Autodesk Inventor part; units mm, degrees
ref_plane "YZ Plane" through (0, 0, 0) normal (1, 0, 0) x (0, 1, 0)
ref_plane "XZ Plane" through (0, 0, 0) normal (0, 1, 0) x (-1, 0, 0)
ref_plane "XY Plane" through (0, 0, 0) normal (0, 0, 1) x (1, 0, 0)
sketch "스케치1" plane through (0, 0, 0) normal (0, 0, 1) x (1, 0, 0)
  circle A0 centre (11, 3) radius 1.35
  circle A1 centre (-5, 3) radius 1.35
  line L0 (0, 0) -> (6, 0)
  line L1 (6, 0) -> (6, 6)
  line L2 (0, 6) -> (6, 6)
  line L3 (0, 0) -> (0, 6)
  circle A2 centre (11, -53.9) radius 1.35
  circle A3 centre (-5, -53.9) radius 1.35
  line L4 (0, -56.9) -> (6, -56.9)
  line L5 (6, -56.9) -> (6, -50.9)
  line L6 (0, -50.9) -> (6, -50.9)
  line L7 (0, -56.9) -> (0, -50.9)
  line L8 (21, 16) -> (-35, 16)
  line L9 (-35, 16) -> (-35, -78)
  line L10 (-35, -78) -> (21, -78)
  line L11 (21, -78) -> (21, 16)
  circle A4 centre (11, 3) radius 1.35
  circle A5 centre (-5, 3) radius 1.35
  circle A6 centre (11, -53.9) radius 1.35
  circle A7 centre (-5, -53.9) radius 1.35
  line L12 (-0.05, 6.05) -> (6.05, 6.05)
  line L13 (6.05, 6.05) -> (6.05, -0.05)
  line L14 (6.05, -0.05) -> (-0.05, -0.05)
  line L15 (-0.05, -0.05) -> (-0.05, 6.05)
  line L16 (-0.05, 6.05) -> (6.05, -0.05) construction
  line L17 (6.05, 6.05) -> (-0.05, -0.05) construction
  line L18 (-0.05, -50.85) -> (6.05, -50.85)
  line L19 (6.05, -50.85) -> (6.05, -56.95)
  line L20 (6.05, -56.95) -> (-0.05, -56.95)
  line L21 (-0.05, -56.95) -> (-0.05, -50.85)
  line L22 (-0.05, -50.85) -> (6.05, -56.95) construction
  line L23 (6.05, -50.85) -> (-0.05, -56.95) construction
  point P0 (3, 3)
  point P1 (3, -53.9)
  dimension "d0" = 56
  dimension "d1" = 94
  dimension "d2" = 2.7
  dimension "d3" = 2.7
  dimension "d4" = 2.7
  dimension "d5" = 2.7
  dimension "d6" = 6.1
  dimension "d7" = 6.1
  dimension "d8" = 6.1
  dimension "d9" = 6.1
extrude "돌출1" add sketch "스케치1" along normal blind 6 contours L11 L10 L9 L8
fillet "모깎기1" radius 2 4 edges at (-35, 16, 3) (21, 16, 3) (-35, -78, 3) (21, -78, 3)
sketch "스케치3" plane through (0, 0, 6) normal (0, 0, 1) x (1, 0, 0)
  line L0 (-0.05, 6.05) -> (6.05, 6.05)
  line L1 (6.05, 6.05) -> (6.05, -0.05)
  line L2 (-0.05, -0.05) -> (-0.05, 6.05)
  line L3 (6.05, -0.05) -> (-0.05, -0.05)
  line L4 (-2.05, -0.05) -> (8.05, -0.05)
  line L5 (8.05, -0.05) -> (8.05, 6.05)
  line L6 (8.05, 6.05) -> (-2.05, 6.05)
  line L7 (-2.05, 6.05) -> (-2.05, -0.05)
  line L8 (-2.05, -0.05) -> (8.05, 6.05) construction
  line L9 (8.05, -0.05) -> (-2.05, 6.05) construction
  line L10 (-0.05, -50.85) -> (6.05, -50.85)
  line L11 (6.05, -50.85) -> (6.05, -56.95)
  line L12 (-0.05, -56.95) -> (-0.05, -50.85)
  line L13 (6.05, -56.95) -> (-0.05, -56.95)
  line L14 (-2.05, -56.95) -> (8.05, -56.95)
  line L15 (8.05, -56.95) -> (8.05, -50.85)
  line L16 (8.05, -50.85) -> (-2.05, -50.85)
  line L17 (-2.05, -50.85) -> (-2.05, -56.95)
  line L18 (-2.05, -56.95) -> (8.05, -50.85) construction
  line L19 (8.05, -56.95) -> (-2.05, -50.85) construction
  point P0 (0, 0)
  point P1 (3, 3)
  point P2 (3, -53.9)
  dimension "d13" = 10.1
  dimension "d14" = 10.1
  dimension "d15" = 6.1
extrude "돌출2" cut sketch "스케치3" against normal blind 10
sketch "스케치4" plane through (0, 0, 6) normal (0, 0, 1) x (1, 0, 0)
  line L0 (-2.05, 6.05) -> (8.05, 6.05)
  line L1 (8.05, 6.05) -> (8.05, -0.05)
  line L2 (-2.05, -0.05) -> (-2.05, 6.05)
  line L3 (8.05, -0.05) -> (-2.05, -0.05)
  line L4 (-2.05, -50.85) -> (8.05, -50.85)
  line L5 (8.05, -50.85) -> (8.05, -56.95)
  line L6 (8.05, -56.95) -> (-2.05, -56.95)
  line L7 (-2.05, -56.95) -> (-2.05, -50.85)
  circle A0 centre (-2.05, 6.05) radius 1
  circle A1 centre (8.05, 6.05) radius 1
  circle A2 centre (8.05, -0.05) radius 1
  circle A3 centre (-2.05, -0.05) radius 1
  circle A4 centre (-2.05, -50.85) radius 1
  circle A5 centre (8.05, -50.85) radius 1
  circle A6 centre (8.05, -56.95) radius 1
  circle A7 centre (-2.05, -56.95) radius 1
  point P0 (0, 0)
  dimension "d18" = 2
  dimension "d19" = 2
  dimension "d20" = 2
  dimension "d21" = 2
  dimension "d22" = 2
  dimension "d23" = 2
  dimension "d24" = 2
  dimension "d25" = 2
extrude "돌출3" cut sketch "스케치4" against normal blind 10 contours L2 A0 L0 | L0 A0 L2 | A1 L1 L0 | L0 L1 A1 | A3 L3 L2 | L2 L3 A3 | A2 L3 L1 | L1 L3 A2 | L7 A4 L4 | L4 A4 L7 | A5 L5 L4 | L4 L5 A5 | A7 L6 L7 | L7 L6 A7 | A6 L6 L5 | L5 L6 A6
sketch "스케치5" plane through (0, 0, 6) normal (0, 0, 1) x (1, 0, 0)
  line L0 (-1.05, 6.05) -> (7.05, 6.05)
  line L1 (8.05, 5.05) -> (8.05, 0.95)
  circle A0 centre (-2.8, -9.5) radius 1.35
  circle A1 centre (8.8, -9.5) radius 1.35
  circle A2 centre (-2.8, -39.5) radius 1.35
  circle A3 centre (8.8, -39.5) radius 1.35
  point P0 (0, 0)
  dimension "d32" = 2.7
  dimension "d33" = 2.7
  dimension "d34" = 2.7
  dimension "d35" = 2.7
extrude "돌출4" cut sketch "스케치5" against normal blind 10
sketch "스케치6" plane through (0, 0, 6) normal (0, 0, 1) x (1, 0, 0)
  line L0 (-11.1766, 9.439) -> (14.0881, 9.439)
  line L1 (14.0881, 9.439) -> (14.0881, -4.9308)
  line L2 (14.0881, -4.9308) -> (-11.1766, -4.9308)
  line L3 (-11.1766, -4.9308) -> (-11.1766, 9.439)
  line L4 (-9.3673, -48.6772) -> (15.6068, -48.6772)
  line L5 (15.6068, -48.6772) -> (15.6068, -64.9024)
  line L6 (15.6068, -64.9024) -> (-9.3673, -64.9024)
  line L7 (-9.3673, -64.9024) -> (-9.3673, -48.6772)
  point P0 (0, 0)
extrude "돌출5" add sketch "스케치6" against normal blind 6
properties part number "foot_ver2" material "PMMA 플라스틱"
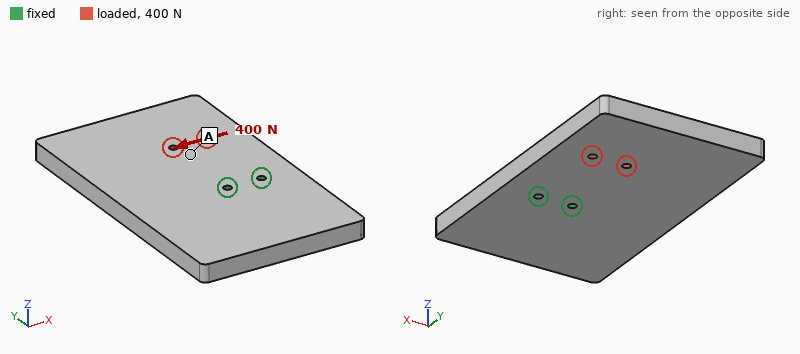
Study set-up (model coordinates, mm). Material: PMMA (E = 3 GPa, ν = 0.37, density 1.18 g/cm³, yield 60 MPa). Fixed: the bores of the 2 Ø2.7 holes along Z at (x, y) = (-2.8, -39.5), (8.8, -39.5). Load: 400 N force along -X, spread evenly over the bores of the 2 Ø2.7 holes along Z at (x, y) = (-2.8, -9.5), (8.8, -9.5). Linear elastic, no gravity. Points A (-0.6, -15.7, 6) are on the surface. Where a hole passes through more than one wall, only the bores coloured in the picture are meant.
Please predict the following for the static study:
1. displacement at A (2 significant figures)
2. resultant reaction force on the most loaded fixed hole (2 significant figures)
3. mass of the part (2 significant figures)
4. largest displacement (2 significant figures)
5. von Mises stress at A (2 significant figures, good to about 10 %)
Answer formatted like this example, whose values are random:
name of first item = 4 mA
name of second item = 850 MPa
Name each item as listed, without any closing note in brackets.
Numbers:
displacement at A = 0.17 mm
resultant reaction force on the most loaded fixed hole = 930 N
mass of the part = 37 g
largest displacement = 0.44 mm
von Mises stress at A = 3.7 MPa
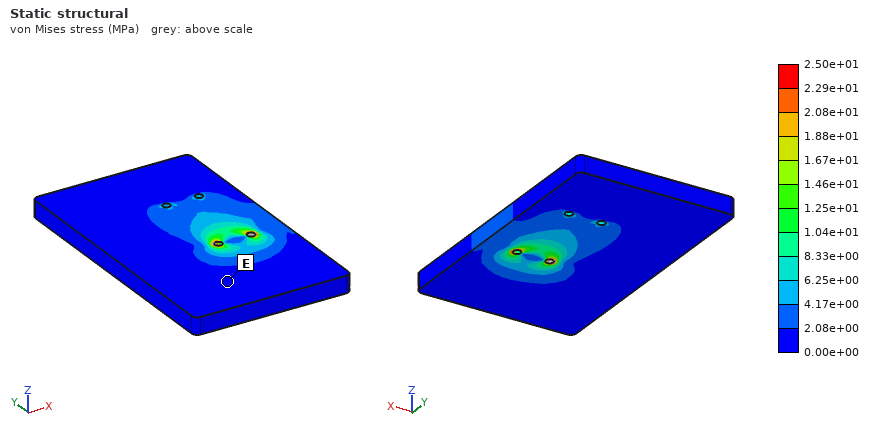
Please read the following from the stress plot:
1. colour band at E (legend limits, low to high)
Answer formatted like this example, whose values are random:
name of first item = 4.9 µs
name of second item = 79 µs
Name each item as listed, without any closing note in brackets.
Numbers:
colour band at E = 0.00e+00 to 2.08e+00 MPa
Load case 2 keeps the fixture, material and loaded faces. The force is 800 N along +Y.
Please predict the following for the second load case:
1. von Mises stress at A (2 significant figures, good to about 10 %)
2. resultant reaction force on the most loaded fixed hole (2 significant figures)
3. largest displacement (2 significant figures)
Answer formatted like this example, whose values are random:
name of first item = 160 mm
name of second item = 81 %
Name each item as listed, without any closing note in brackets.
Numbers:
von Mises stress at A = 4.9 MPa
resultant reaction force on the most loaded fixed hole = 400 N
largest displacement = 57 µm
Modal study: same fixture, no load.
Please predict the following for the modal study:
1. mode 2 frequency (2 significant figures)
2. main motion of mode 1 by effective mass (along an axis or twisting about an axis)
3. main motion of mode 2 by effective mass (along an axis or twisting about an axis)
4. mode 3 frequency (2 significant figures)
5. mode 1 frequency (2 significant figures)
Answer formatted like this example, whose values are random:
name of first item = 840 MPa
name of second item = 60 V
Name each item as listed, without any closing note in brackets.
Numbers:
mode 2 frequency = 820 Hz
main motion of mode 1 by effective mass = along Z
main motion of mode 2 by effective mass = along Z
mode 3 frequency = 890 Hz
mode 1 frequency = 410 Hz
